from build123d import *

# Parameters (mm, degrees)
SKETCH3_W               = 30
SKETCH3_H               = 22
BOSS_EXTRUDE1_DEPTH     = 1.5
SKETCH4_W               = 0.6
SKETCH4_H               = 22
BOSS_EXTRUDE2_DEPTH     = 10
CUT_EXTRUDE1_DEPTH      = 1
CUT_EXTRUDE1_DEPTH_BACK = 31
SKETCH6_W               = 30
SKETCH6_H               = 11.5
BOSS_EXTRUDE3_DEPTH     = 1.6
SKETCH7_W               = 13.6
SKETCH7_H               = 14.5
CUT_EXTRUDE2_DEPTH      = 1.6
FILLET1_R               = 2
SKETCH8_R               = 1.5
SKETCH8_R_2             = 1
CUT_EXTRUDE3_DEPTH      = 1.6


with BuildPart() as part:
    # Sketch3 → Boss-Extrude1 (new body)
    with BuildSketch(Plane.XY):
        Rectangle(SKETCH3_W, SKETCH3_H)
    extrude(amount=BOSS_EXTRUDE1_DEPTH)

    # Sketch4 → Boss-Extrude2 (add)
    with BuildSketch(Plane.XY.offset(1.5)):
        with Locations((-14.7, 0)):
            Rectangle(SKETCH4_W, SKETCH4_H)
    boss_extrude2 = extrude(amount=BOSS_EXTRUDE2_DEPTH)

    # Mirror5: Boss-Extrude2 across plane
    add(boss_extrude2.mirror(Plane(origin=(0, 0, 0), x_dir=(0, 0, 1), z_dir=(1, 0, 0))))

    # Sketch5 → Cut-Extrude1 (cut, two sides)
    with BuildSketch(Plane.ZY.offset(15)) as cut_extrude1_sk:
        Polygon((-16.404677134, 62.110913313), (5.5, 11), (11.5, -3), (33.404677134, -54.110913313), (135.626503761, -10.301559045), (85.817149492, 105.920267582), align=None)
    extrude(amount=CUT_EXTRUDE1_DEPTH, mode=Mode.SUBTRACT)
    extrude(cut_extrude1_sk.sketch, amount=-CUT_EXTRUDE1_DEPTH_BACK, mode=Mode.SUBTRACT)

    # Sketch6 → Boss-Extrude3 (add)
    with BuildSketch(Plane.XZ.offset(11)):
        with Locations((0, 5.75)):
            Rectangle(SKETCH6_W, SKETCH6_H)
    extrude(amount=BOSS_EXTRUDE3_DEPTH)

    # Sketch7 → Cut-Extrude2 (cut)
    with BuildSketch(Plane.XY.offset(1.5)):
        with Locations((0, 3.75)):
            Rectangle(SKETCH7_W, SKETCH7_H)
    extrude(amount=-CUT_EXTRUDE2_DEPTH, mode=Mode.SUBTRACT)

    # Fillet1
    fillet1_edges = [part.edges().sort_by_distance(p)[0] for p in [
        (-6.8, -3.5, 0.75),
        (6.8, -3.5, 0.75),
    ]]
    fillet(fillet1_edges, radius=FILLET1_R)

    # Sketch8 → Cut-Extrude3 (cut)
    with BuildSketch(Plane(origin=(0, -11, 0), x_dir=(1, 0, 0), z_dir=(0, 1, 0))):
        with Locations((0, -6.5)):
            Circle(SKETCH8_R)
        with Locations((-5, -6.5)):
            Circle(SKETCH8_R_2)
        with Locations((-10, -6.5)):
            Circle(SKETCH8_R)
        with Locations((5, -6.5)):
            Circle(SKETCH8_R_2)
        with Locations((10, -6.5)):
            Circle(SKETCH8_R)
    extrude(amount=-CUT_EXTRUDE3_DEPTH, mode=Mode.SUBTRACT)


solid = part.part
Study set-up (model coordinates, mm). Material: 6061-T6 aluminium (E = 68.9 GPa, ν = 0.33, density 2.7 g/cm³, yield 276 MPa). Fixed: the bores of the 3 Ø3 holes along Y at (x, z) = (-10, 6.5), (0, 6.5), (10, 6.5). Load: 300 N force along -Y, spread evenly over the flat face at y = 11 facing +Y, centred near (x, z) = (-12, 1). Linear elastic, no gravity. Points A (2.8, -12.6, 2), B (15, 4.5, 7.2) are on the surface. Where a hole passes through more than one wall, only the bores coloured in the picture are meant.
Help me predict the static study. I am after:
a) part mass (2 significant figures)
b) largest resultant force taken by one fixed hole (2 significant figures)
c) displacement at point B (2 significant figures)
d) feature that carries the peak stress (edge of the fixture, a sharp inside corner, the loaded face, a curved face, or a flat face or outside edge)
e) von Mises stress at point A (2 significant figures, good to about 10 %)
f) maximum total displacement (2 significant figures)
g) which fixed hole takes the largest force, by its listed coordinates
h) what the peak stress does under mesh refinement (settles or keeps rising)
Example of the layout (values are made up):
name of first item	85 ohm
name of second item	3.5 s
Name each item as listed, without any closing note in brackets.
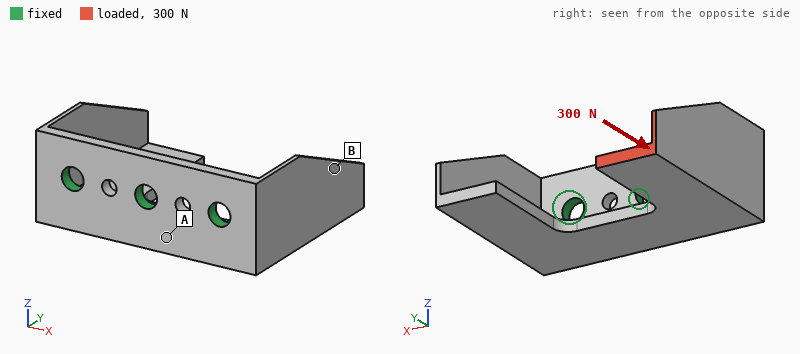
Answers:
part mass	3.8 g
largest resultant force taken by one fixed hole	270 N
displacement at point B	0.035 mm
feature that carries the peak stress	edge of the fixture
von Mises stress at point A	30 MPa
maximum total displacement	0.15 mm
which fixed hole takes the largest force, by its listed coordinates	(-10, 6.5)
what the peak stress does under mesh refinement	keeps rising
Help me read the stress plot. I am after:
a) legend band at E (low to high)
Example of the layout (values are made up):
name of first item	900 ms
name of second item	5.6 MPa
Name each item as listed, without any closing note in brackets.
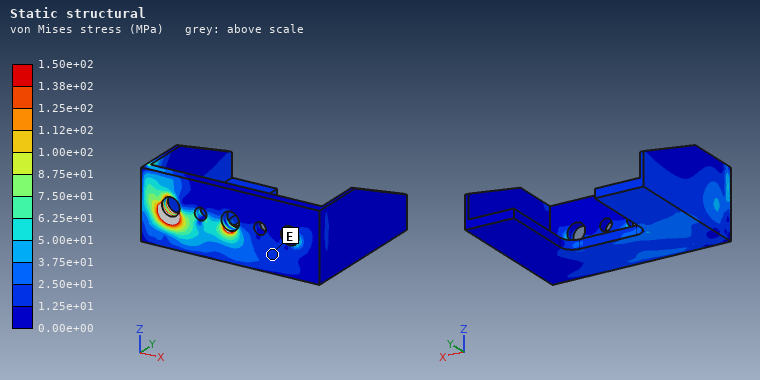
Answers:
legend band at E	1.25e+01 to 2.50e+01 MPa
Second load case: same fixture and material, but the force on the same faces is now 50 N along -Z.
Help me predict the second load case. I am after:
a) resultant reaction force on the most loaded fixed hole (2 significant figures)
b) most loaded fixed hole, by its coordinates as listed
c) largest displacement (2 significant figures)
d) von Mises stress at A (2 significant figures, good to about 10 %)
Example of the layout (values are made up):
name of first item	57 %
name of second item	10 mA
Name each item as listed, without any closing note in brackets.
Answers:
resultant reaction force on the most loaded fixed hole	62 N
most loaded fixed hole, by its coordinates as listed	(-10, 6.5)
largest displacement	0.24 mm
von Mises stress at A	24 MPa
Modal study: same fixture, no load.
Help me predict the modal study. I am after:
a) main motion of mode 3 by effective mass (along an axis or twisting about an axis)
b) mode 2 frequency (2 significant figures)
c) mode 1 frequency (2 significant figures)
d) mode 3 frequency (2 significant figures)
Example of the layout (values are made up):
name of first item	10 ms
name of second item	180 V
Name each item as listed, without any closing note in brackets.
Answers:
main motion of mode 3 by effective mass	along X
mode 2 frequency	4400 Hz
mode 1 frequency	4300 Hz
mode 3 frequency	7600 Hz
